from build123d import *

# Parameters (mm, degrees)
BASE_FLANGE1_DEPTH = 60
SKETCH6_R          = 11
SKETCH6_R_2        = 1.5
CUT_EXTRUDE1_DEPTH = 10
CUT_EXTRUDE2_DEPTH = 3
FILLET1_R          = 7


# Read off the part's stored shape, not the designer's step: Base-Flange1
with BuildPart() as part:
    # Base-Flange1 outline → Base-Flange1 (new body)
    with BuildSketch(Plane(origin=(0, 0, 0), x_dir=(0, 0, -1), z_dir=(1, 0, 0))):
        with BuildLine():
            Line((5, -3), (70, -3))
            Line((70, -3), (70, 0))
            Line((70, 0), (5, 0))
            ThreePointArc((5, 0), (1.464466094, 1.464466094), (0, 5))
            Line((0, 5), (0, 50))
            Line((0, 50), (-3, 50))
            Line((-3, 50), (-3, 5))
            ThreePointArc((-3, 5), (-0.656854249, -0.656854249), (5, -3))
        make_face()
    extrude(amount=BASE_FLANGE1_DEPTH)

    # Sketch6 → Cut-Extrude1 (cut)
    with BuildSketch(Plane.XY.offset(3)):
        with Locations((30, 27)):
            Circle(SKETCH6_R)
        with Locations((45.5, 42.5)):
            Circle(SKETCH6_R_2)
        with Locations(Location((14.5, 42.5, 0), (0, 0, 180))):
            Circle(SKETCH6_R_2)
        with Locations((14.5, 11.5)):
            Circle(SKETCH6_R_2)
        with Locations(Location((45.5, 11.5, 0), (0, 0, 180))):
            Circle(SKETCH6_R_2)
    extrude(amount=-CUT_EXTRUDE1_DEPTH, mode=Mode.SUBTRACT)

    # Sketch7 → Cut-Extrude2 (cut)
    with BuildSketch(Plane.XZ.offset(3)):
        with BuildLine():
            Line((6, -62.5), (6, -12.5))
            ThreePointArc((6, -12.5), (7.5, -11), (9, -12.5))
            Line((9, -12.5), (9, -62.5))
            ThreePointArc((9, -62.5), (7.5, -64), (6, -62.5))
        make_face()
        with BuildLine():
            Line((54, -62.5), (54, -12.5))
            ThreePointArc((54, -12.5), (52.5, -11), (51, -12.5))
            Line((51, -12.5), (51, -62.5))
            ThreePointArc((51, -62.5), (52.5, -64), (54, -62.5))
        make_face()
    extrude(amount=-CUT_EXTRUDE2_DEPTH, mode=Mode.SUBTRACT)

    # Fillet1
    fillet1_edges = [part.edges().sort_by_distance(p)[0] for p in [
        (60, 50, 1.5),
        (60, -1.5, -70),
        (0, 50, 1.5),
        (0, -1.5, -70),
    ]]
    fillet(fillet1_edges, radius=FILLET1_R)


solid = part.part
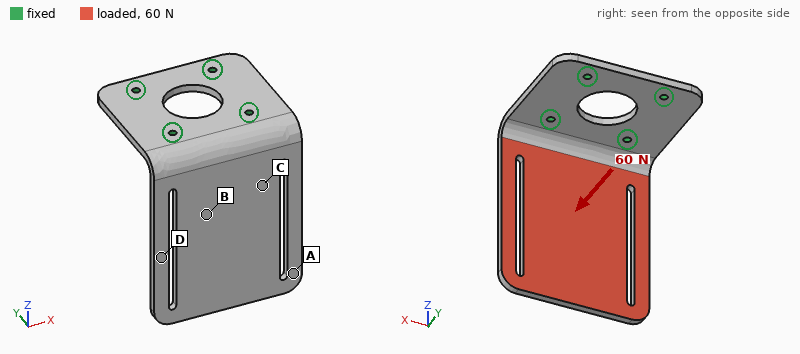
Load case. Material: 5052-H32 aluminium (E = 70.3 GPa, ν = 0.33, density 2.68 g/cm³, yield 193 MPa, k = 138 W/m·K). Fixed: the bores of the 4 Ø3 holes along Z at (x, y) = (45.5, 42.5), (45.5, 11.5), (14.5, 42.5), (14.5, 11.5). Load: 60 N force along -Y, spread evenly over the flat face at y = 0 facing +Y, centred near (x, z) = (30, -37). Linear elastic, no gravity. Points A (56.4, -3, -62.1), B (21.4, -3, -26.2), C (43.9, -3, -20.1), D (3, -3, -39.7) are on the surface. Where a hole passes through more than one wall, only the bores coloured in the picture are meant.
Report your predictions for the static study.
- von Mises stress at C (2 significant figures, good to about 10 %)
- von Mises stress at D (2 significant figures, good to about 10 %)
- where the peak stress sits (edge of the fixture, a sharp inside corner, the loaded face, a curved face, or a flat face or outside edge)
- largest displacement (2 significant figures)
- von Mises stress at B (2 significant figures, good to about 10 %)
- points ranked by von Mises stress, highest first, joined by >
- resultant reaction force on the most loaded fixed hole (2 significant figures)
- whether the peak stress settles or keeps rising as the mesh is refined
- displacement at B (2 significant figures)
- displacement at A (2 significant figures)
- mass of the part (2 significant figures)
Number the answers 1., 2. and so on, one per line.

1. 13 MPa
2. 5.7 MPa
3. edge of the fixture
4. 0.52 mm
5. 10.0 MPa
6. C > B > D > A
7. 32 N
8. keeps rising
9. 0.15 mm
10. 0.44 mm
11. 52 g
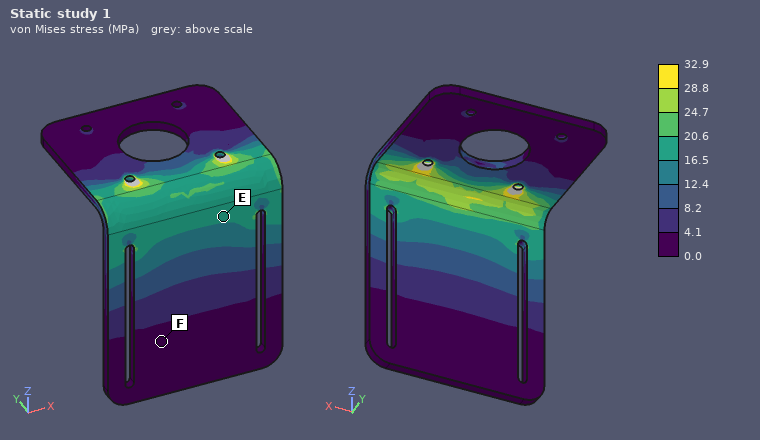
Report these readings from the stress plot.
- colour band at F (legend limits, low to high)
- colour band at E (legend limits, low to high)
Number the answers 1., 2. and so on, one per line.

1. 0.0 to 4.1 MPa
2. 16.5 to 20.6 MPa
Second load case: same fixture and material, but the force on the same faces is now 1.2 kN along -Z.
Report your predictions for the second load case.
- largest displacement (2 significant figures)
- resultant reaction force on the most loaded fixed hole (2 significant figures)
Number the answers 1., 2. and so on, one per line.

1. 0.46 mm
2. 660 N
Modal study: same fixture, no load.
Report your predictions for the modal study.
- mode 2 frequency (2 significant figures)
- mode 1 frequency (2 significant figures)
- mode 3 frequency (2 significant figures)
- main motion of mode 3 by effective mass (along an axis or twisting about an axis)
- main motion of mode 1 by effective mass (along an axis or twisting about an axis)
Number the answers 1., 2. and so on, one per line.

1. 1100 Hz
2. 400 Hz
3. 1700 Hz
4. along X
5. along Y
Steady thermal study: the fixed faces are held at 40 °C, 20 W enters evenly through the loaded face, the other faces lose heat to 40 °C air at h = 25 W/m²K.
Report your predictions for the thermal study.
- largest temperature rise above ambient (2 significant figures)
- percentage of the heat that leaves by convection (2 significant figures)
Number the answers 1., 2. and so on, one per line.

1. 37 K
2. 21 %
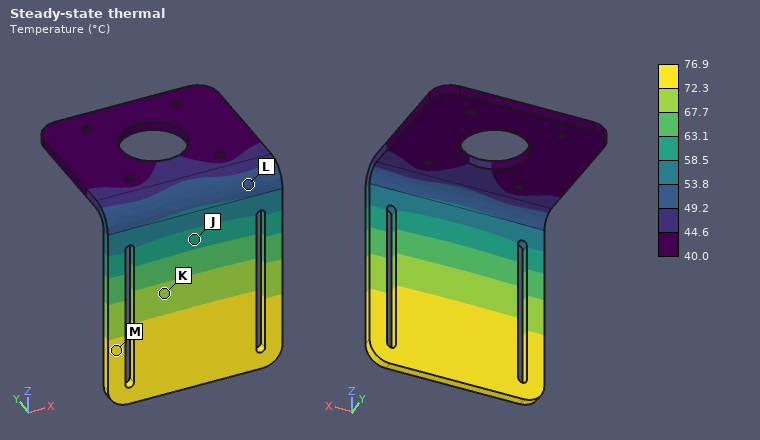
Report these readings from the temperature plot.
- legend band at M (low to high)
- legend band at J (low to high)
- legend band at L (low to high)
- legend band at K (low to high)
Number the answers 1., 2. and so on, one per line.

1. 72.3 to 76.9 °C
2. 58.5 to 63.1 °C
3. 49.2 to 53.8 °C
4. 67.7 to 72.3 °C
